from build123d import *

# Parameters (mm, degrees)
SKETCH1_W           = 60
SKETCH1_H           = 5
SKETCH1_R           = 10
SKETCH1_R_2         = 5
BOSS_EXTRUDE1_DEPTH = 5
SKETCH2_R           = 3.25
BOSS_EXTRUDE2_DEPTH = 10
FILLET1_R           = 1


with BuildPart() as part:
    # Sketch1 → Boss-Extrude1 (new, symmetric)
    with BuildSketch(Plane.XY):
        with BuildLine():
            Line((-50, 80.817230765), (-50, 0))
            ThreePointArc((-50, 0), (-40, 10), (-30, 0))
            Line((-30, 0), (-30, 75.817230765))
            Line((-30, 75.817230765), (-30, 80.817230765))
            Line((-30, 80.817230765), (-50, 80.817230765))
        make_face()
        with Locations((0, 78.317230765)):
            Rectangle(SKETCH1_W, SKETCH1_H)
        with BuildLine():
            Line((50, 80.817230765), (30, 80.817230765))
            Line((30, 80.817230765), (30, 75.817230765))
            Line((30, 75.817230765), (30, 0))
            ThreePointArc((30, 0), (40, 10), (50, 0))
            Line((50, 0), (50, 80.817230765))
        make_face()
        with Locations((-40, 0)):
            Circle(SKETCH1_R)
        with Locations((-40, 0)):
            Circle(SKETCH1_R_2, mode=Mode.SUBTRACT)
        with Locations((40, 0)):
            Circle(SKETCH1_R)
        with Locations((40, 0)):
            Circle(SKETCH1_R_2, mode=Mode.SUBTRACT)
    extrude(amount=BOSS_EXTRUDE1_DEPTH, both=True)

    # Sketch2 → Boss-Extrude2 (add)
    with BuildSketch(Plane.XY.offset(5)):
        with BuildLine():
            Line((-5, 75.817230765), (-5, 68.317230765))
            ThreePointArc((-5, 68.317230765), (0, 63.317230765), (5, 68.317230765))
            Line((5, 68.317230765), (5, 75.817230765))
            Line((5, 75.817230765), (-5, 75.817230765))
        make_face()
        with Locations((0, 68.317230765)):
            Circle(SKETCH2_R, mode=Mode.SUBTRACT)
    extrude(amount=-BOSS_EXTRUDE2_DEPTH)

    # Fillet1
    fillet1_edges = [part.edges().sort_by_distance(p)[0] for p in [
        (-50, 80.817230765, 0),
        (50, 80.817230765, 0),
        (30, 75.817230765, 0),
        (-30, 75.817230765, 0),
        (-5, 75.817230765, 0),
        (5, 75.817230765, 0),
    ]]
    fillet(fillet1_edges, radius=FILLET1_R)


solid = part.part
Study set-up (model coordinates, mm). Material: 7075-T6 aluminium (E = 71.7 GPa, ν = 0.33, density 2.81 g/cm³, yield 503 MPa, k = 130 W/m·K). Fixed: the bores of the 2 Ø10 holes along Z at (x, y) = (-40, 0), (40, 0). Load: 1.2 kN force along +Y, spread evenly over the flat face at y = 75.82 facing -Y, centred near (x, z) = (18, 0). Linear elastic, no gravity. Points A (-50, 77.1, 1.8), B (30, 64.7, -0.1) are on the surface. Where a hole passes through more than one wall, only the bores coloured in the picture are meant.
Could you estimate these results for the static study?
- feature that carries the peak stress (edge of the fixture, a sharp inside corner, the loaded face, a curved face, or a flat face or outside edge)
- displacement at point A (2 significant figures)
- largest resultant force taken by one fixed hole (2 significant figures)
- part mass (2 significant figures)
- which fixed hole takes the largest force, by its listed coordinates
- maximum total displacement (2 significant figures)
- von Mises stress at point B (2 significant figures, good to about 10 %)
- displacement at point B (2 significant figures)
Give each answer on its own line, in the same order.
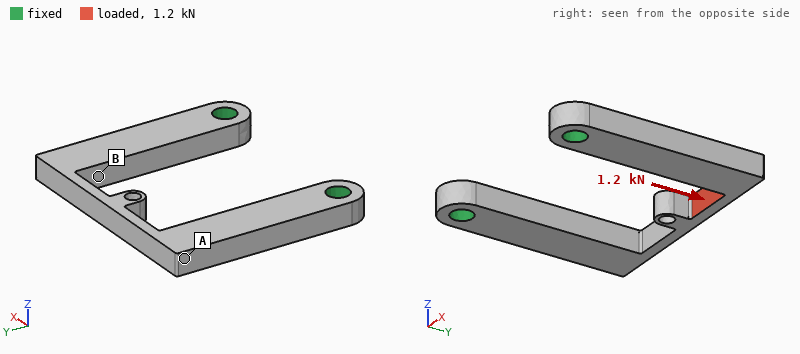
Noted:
a curved face
0.034 mm
1.0 kN
110 g
(40, 0)
0.14 mm
25 MPa
0.024 mm
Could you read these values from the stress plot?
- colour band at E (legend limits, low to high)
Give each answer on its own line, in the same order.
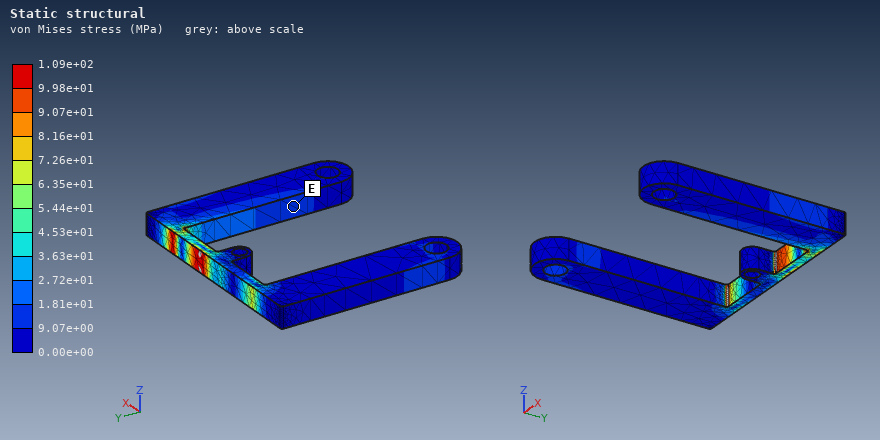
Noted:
9.07e+00 to 1.81e+01 MPa
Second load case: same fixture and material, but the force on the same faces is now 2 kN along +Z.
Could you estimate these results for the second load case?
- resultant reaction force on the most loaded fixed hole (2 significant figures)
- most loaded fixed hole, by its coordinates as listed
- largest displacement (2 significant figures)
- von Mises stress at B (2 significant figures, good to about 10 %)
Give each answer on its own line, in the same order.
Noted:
1.3 kN
(40, 0)
1.6 mm
43 MPa
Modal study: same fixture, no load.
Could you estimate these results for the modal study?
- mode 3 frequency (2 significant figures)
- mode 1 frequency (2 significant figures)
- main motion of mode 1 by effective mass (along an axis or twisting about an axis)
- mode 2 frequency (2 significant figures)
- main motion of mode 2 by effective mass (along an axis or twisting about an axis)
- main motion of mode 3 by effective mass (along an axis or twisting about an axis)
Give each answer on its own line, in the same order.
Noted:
2000 Hz
1100 Hz
along Z
1800 Hz
twisting about Y
along X
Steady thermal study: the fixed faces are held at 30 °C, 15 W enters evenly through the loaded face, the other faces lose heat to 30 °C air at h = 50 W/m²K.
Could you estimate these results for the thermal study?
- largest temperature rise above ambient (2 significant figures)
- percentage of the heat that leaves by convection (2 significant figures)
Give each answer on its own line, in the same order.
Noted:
36 K
41 %
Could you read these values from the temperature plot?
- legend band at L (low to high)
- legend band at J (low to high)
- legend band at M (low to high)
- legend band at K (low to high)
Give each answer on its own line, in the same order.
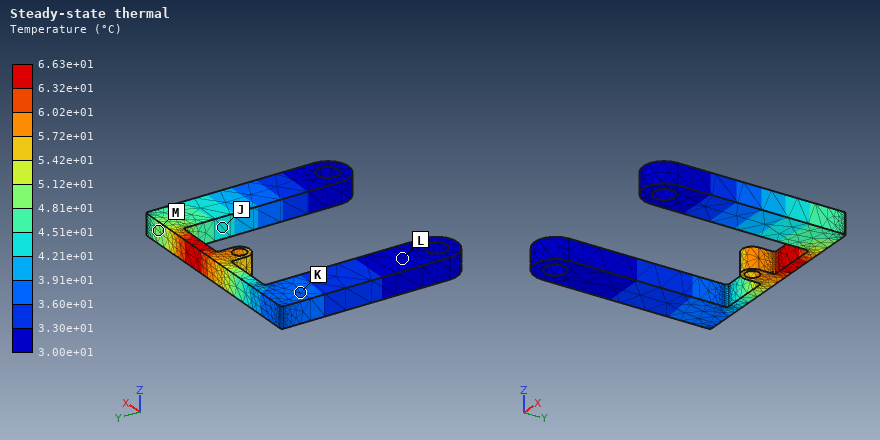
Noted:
3.00e+01 to 3.30e+01 °C
4.21e+01 to 4.51e+01 °C
4.81e+01 to 5.12e+01 °C
3.60e+01 to 3.91e+01 °C
